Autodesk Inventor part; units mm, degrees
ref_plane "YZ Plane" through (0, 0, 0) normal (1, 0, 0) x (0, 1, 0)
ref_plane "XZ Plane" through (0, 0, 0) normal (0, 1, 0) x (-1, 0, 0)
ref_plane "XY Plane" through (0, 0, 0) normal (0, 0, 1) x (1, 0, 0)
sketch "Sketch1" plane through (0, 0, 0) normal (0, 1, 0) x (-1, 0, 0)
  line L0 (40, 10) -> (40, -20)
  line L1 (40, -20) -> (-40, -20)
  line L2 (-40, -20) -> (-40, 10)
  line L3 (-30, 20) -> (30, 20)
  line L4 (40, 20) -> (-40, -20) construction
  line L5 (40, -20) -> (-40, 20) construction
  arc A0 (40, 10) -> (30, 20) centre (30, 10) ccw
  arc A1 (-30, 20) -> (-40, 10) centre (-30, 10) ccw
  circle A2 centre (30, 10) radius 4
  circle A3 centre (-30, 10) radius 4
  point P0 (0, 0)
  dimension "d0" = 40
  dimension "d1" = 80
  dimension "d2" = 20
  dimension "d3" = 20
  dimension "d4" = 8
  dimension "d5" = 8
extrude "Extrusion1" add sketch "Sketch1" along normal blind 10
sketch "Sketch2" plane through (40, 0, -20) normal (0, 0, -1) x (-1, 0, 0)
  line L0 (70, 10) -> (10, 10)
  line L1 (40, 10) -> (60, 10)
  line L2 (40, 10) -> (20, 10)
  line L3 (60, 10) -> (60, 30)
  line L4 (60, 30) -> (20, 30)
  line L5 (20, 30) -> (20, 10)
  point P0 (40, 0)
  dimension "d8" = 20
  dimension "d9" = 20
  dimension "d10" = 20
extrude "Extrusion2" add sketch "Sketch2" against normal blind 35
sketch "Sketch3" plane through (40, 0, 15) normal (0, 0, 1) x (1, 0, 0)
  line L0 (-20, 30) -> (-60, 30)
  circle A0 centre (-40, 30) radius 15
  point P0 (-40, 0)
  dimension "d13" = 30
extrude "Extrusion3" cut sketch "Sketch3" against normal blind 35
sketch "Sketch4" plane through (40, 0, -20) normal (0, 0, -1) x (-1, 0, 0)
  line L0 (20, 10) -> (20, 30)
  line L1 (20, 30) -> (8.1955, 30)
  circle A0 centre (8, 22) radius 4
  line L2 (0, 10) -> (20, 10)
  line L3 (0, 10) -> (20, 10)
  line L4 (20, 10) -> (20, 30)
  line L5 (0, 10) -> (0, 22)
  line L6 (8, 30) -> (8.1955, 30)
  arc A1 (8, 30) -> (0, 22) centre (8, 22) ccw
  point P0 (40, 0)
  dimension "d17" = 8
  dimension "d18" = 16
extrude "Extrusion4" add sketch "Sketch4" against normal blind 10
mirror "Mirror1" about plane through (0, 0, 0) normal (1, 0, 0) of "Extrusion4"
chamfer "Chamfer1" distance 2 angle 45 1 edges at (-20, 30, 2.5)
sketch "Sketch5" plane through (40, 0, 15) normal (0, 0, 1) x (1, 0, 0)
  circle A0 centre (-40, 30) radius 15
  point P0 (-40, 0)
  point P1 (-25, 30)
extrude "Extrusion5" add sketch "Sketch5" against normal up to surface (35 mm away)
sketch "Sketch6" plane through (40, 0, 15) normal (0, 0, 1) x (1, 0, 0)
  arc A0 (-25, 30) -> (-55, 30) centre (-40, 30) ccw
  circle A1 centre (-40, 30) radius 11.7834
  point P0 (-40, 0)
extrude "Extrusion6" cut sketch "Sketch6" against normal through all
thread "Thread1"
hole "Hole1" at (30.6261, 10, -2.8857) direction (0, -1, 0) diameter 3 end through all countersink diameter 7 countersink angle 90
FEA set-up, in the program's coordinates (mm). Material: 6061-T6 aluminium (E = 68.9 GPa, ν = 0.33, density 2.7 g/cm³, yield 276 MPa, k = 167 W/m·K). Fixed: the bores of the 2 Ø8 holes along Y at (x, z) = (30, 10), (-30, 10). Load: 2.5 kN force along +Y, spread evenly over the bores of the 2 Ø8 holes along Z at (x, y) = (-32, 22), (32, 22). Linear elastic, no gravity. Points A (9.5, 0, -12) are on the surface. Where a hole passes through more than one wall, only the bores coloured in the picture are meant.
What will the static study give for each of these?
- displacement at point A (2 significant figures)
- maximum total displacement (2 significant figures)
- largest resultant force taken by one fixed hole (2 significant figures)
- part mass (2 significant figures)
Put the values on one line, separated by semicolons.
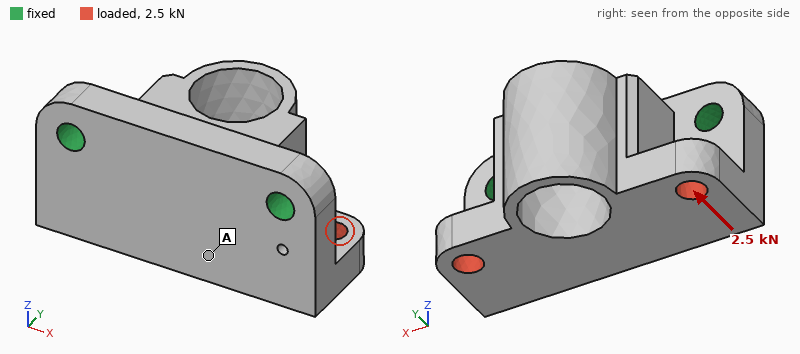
29 µm; 64 µm; 1.3 kN; 170 g
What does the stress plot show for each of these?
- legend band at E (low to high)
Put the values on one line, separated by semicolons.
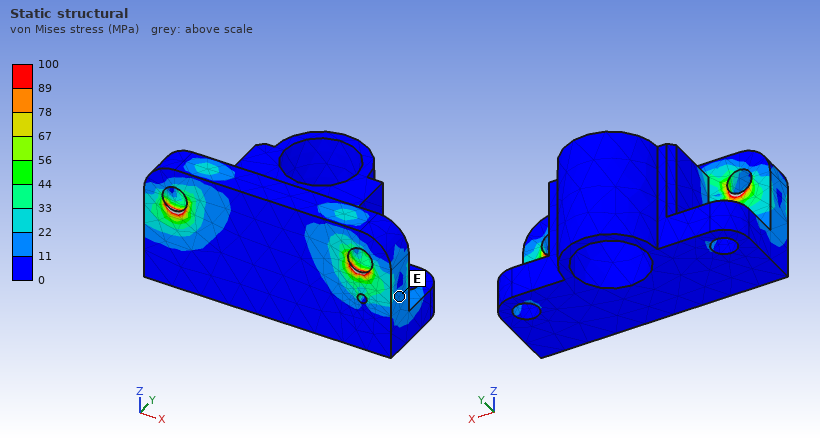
11 to 22 MPa
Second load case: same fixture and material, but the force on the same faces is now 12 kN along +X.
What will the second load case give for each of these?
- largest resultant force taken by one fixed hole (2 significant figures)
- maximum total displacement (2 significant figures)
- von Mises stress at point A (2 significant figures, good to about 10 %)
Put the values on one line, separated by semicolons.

8.5 kN; 57 µm; 12 MPa
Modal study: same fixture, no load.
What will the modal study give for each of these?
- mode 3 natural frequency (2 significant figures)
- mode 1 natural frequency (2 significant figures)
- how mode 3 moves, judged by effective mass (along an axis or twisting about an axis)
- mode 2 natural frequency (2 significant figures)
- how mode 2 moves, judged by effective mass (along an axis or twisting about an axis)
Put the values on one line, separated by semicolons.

11 kHz; 3700 Hz; along Y; 8700 Hz; along X
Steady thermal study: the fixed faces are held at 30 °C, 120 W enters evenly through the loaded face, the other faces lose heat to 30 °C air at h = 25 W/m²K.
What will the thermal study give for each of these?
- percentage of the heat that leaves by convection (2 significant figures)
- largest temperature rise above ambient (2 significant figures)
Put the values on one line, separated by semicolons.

5.8 %; 47 K
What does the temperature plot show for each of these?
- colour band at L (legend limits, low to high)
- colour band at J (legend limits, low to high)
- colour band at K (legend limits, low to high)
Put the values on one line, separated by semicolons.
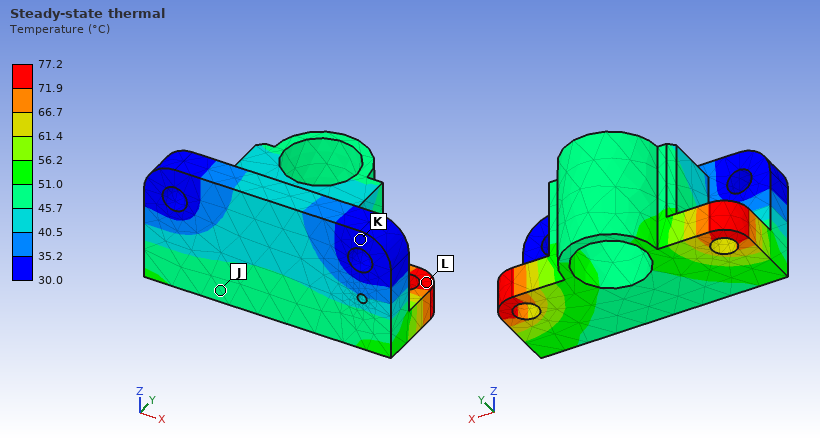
71.9 to 77.2 °C; 45.7 to 51.0 °C; 30.0 to 35.2 °C
